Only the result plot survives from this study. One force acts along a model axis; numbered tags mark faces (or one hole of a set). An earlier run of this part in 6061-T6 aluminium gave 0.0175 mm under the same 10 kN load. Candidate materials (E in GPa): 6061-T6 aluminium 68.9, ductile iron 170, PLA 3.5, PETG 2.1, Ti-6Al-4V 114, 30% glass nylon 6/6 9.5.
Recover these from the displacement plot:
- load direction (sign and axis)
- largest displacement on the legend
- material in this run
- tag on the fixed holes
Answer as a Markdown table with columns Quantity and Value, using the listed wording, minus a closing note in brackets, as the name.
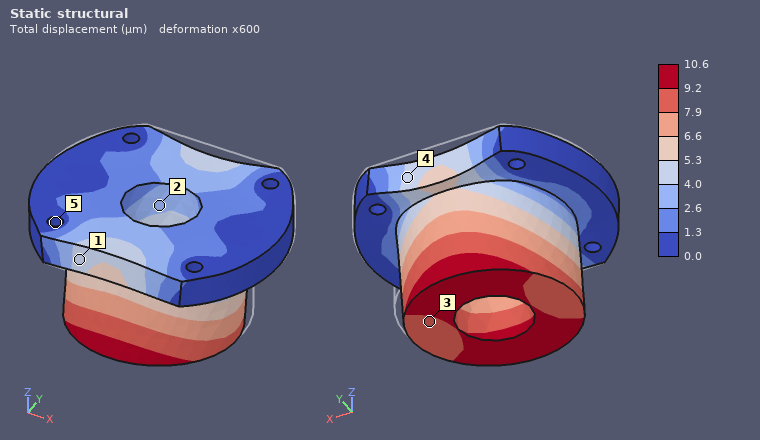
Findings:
| Quantity | Value |
|---|---|
| load direction | -Y |
| largest displacement on the legend | 10.6 µm |
| material in this run | Ti-6Al-4V |
| tag on the fixed holes | 5 |
